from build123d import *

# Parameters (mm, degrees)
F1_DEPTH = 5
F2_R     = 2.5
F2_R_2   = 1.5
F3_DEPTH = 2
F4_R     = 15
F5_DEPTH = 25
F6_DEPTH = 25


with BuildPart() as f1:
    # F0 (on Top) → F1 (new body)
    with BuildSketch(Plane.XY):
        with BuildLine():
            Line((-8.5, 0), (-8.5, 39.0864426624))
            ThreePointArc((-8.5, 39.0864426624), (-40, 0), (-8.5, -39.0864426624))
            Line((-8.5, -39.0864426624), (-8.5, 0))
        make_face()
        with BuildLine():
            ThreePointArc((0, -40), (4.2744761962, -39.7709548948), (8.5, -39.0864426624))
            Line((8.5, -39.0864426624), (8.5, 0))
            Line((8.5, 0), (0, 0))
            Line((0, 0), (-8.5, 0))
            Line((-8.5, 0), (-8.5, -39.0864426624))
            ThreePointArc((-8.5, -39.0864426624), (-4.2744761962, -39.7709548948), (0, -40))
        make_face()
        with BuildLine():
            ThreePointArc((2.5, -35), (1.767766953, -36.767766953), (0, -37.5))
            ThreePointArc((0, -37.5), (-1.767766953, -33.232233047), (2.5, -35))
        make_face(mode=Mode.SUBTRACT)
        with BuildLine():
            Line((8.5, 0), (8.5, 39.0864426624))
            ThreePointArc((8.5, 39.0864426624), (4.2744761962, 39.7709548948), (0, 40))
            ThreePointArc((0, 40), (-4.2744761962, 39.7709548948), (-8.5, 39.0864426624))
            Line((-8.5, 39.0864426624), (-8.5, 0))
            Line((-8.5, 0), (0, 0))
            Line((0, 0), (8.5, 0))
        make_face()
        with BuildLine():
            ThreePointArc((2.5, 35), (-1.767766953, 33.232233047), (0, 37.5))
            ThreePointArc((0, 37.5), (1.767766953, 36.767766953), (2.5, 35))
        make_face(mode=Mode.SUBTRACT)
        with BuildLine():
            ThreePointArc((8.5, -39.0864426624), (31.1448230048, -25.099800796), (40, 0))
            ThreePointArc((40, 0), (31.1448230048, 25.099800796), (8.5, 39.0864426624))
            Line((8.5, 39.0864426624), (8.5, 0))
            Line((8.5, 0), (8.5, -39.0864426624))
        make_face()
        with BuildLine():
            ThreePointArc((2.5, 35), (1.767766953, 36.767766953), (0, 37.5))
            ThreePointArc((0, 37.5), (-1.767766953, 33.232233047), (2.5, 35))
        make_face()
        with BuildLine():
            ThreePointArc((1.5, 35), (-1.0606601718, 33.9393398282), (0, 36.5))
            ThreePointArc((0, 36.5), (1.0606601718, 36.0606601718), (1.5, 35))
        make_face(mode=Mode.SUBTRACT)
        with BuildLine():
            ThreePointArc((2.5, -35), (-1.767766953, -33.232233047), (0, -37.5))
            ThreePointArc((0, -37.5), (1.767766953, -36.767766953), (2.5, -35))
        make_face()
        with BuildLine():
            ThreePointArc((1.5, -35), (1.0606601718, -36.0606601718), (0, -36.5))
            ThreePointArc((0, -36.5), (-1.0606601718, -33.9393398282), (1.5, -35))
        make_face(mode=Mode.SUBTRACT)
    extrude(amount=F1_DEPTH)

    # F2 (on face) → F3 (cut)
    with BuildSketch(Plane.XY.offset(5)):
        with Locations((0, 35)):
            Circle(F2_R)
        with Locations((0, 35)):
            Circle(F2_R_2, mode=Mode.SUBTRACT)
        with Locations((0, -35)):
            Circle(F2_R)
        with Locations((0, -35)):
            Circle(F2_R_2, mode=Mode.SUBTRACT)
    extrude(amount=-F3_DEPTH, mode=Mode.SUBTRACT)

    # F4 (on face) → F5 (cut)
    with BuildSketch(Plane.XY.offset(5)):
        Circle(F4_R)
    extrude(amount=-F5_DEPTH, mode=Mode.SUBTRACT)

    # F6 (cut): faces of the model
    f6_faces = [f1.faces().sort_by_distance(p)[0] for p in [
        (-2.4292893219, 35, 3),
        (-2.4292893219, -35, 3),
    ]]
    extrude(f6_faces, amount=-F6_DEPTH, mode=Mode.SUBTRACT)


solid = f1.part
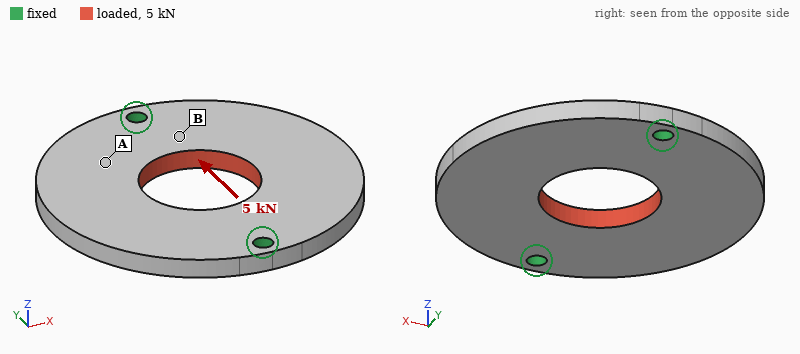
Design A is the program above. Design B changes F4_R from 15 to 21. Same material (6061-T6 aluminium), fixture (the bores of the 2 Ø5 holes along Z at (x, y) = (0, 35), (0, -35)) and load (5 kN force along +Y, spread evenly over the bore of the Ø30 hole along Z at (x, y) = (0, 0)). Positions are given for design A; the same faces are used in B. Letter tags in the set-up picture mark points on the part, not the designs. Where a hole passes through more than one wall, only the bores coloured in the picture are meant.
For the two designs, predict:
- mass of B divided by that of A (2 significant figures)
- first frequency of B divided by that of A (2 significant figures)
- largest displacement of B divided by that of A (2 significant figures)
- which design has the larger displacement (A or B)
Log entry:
0.84
0.99
1.5
B
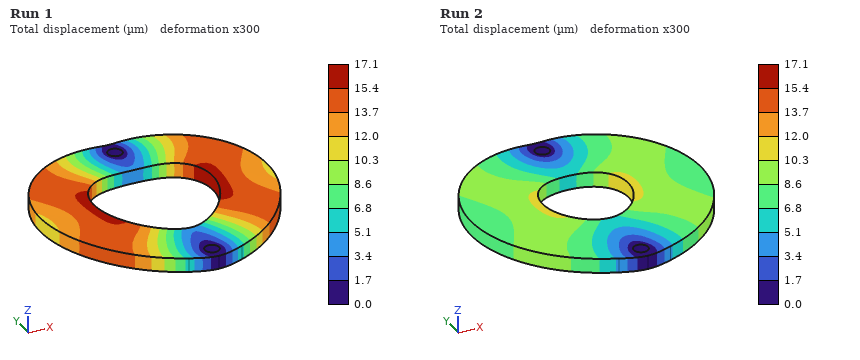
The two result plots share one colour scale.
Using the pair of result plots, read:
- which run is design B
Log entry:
Run 1
